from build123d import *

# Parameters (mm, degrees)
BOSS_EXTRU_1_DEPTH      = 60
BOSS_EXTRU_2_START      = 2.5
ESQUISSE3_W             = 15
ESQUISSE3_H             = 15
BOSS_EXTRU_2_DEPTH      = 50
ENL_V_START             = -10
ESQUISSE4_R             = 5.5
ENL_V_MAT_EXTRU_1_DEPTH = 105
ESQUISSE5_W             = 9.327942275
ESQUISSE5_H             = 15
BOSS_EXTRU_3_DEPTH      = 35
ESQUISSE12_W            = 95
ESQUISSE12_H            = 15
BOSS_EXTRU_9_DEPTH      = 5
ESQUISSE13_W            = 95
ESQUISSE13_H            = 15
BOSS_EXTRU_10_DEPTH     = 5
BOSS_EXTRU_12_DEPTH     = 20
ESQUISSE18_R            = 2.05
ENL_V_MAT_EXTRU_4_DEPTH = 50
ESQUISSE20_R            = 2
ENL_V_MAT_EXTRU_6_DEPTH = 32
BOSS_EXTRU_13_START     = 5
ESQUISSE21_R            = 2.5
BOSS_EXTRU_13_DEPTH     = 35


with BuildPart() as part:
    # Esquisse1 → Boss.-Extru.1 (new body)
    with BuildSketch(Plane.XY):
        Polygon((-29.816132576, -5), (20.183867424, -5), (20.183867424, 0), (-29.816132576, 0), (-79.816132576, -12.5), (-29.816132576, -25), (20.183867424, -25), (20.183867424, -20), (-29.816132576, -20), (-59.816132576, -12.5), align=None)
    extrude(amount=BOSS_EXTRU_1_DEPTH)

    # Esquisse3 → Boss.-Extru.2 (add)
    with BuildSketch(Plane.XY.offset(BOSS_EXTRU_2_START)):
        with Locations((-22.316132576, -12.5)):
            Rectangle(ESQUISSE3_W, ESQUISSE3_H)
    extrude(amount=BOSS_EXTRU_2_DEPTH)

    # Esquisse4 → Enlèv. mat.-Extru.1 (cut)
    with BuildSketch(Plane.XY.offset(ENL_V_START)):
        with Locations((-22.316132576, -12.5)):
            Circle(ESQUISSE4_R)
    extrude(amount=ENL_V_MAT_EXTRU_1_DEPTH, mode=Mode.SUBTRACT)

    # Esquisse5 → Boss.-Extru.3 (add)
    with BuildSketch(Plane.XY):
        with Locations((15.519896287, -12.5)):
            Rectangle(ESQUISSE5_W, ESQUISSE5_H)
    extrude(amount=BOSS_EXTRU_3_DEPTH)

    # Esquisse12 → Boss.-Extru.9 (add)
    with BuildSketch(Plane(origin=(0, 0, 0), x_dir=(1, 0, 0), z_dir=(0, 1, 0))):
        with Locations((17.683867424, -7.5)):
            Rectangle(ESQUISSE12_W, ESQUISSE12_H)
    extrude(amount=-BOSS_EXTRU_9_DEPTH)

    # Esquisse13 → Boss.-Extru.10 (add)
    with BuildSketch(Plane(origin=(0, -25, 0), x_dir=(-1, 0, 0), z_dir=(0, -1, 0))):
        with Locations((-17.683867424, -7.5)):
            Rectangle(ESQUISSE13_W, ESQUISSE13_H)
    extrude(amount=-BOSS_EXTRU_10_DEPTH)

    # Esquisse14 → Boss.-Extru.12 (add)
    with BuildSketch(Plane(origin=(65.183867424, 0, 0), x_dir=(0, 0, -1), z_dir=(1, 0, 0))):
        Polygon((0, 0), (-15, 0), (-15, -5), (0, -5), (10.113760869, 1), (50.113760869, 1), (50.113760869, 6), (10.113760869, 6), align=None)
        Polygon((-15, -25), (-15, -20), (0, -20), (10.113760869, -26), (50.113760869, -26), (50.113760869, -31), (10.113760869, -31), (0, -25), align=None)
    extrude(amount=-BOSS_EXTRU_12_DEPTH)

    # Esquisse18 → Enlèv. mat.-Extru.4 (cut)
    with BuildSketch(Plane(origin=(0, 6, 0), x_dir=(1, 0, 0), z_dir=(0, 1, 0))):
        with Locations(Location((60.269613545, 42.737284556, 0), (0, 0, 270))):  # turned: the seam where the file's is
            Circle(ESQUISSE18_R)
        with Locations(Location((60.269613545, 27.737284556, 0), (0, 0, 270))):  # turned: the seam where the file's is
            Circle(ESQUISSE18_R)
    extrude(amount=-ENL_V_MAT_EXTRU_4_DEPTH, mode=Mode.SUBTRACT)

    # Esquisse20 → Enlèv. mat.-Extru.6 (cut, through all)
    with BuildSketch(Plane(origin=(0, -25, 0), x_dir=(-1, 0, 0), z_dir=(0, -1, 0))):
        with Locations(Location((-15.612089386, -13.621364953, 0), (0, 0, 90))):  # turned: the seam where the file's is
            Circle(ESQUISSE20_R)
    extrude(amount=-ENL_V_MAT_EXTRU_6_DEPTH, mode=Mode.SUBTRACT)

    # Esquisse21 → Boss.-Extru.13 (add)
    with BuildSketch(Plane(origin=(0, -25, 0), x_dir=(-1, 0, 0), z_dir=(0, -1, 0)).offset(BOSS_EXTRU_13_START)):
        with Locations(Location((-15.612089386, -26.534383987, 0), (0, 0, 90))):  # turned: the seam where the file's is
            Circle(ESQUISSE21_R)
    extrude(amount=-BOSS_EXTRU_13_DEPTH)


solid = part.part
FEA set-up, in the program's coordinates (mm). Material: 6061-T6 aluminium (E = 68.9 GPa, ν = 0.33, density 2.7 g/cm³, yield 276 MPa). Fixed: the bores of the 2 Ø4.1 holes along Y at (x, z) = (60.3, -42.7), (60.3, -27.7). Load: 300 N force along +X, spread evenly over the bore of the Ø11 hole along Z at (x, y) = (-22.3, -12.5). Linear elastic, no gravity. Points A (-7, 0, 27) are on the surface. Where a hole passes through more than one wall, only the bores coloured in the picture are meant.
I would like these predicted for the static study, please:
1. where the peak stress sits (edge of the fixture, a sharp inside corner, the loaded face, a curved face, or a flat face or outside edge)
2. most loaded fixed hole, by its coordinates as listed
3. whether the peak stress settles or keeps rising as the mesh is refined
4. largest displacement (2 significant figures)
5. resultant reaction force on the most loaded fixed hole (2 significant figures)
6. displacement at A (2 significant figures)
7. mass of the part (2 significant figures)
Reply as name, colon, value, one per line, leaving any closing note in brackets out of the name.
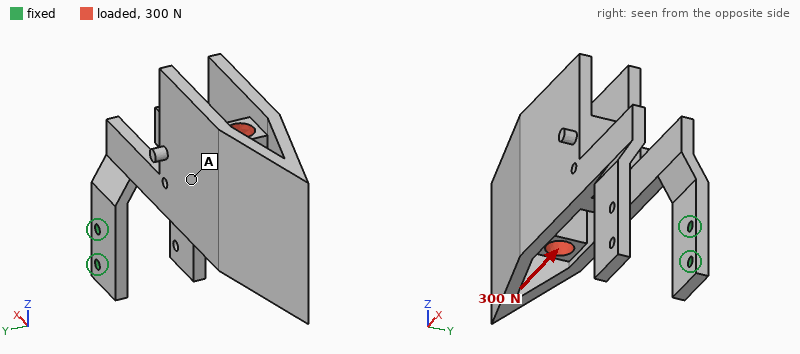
where the peak stress sits: edge of the fixture
most loaded fixed hole, by its coordinates as listed: (60.3, -27.7)
whether the peak stress settles or keeps rising as the mesh is refined: keeps rising
largest displacement: 1.9 mm
resultant reaction force on the most loaded fixed hole: 1.2 kN
displacement at A: 0.76 mm
mass of the part: 220 g
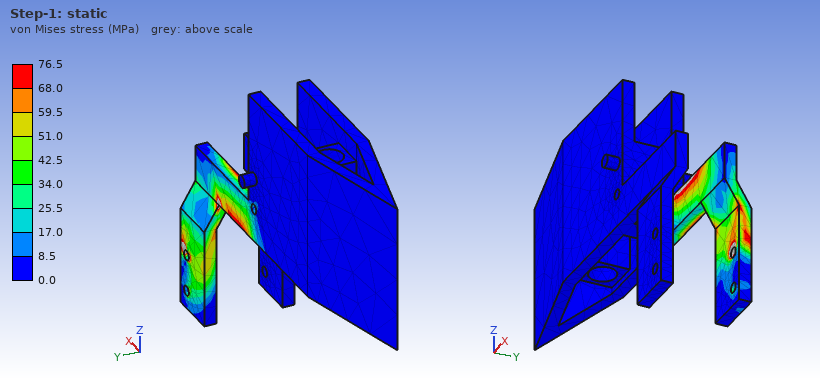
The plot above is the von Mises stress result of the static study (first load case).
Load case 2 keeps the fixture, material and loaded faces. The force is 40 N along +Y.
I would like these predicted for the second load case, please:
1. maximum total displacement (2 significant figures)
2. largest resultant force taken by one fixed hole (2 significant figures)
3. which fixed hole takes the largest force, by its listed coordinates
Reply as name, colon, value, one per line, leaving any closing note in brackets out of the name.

maximum total displacement: 2.1 mm
largest resultant force taken by one fixed hole: 110 N
which fixed hole takes the largest force, by its listed coordinates: (60.3, -27.7)
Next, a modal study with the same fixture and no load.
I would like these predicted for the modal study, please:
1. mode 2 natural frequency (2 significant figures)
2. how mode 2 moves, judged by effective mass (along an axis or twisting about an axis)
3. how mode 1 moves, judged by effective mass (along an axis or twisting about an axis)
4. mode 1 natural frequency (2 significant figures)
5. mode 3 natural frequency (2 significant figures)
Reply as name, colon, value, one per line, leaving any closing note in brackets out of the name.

mode 2 natural frequency: 170 Hz
how mode 2 moves, judged by effective mass: along Z
how mode 1 moves, judged by effective mass: along Y
mode 1 natural frequency: 66 Hz
mode 3 natural frequency: 250 Hz
